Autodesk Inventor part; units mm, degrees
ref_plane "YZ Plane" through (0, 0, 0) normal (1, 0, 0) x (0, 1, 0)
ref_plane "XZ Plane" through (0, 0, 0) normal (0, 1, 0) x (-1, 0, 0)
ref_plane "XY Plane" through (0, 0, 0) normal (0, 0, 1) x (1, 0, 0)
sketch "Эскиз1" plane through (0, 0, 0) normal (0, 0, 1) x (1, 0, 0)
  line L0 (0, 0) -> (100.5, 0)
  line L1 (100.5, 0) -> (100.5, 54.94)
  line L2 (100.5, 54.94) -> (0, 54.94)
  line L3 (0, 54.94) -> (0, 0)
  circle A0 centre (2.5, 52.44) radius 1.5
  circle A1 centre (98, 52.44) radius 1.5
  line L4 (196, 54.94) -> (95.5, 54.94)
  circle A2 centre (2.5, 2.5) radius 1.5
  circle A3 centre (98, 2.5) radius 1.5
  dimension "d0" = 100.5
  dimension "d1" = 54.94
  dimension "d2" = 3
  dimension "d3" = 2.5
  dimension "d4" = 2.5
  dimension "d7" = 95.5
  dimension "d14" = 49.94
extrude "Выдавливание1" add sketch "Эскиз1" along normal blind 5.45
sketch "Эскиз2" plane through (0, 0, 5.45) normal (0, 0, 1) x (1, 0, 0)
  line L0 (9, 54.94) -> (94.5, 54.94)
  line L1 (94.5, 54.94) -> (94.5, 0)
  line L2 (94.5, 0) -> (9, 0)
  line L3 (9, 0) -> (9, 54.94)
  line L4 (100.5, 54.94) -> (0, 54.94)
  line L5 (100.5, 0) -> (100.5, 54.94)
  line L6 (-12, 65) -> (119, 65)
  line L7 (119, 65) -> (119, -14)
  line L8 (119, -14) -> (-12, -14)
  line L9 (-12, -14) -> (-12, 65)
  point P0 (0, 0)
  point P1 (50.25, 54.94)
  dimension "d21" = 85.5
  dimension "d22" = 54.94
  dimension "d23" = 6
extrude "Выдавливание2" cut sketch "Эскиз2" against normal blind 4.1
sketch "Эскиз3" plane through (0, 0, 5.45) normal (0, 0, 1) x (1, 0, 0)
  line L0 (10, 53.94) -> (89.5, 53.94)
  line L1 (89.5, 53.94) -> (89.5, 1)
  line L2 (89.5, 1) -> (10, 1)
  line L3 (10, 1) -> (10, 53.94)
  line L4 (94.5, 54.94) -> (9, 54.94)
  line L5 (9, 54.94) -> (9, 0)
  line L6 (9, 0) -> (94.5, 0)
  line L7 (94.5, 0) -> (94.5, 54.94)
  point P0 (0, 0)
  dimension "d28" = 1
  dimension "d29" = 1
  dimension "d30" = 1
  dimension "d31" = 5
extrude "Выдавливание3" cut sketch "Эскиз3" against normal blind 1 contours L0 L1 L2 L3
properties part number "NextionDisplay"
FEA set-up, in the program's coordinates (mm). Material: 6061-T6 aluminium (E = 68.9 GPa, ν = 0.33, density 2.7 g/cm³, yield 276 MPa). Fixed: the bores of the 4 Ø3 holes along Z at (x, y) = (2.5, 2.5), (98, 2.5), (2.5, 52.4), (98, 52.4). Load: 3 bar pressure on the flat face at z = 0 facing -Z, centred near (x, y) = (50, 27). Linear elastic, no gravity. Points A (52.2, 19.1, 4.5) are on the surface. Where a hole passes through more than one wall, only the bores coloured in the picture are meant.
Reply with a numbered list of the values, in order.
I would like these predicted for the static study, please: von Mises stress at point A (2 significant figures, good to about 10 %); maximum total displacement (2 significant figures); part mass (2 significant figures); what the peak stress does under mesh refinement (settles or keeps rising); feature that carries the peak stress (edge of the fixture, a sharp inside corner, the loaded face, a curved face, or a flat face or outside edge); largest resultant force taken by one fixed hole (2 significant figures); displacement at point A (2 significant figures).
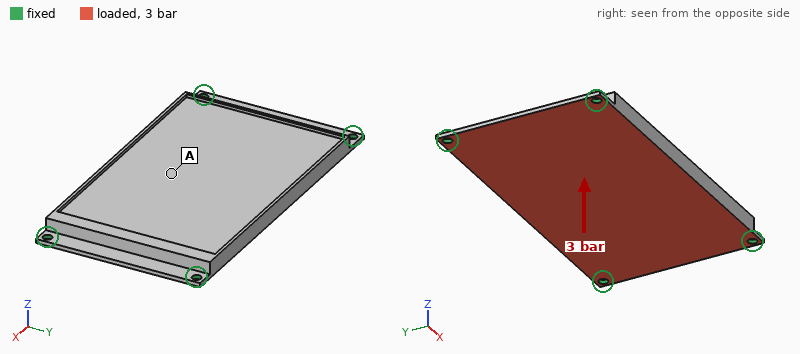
1. 65 MPa
2. 0.38 mm
3. 61 g
4. keeps rising
5. edge of the fixture
6. 1.3 kN
7. 0.37 mm
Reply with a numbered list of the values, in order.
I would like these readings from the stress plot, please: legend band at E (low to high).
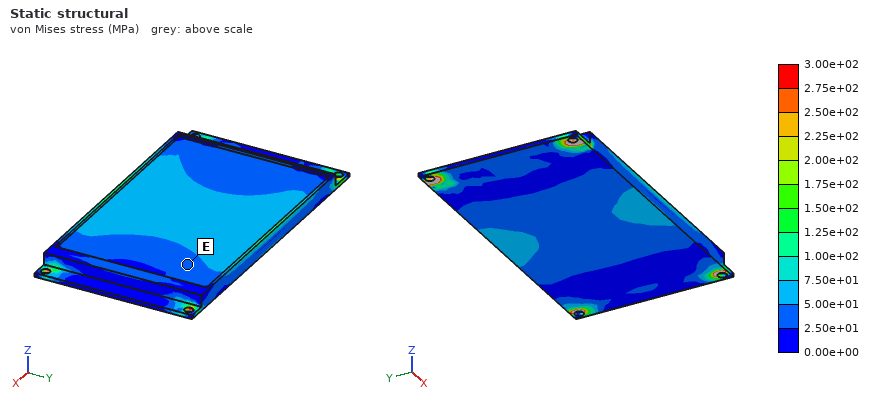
1. 2.50e+01 to 5.00e+01 MPa
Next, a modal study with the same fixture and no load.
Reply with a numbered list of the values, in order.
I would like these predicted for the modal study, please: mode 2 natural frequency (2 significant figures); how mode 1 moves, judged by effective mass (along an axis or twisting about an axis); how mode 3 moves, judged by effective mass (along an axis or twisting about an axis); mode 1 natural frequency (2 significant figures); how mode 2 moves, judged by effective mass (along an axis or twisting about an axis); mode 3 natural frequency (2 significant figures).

1. 2800 Hz
2. along Z
3. twisting about Y
4. 1500 Hz
5. twisting about X
6. 3800 Hz
